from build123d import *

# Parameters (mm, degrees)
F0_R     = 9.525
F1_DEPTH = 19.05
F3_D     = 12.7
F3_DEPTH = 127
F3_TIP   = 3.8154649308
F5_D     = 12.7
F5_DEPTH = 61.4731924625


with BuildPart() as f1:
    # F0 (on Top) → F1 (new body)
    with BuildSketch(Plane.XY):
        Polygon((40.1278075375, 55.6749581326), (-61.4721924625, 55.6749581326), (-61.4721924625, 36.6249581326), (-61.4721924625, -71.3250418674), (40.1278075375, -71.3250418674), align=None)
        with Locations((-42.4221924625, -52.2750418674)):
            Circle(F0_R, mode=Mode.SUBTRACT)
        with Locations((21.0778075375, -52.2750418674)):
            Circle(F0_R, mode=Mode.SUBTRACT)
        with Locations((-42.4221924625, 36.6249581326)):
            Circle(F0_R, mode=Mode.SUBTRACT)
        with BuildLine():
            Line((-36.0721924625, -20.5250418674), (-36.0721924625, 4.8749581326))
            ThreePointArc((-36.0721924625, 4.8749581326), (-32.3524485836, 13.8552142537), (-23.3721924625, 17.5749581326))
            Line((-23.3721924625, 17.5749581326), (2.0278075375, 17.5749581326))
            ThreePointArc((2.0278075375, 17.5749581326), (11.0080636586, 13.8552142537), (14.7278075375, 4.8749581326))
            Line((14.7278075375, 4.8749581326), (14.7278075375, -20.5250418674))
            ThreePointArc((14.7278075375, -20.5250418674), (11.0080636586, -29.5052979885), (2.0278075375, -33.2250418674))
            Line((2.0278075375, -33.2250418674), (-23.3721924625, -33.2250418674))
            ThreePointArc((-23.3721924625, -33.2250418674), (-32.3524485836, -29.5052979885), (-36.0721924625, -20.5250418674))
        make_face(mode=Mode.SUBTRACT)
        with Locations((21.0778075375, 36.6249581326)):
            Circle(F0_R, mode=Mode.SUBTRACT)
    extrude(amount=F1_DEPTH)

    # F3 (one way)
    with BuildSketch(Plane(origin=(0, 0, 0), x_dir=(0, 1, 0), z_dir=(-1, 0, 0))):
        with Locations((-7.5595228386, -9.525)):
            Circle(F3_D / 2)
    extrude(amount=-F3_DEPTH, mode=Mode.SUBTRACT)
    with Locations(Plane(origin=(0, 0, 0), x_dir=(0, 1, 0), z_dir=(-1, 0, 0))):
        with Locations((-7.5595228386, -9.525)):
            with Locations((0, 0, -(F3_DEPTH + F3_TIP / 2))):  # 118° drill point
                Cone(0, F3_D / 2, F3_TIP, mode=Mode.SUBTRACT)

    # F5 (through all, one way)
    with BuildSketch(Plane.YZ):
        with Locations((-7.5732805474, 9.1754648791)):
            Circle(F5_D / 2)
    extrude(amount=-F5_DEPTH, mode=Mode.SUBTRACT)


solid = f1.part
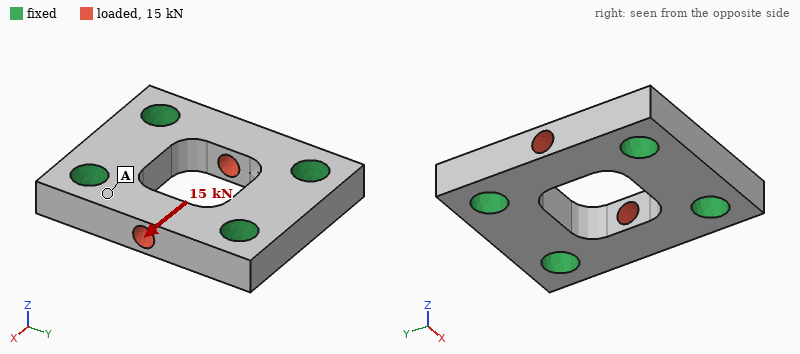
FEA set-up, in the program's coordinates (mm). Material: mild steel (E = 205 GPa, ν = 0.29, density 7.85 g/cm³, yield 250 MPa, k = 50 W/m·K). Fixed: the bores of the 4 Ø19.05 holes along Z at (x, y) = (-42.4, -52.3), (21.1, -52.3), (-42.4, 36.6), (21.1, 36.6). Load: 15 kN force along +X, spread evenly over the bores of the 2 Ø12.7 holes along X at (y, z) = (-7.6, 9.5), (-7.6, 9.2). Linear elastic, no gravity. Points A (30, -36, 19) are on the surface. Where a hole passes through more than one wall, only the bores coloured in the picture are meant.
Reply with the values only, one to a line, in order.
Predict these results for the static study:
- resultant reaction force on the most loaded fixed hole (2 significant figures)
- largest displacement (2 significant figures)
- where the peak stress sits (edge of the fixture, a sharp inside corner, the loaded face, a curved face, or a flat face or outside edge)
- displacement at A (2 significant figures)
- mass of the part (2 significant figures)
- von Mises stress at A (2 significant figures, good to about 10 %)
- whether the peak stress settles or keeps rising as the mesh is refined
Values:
3.8 kN
6.6 µm
a sharp inside corner
1.2 µm
1.3 kg
8.9 MPa
keeps rising
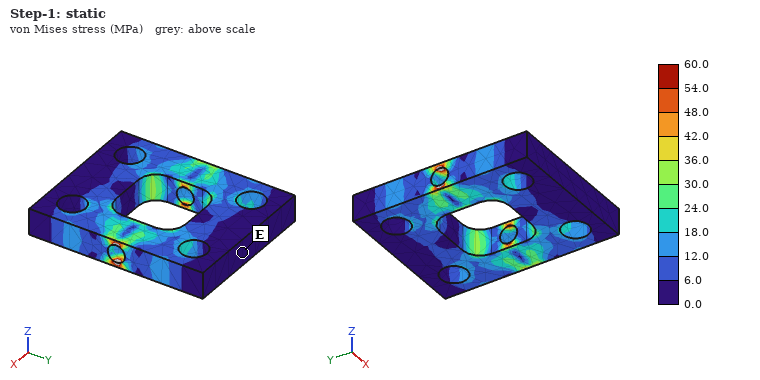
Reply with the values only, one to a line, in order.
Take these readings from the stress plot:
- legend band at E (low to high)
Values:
0.0 to 6.0 MPa
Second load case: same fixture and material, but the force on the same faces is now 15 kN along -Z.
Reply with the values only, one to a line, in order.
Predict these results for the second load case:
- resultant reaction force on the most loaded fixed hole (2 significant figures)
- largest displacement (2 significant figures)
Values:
3.8 kN
10 µm
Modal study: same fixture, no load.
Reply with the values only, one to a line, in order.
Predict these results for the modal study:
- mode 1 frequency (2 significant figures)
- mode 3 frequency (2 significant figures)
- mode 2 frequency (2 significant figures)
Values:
15 kHz
18 kHz
15 kHz
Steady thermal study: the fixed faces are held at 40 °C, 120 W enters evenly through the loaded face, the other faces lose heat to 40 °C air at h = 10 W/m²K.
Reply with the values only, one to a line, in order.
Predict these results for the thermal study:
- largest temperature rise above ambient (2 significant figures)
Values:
41 K
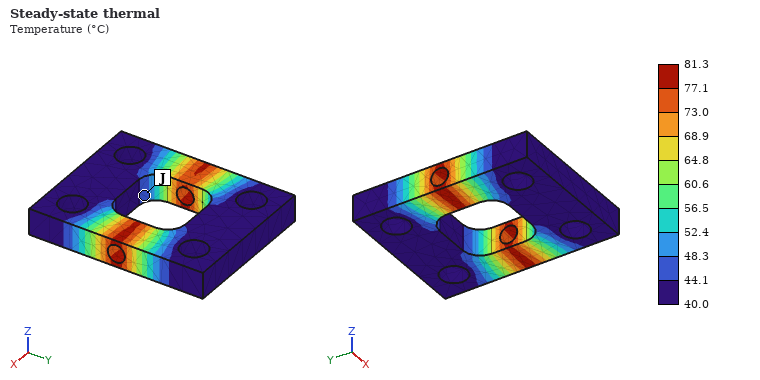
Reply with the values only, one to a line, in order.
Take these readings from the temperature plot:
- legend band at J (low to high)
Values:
44.1 to 48.3 °C
